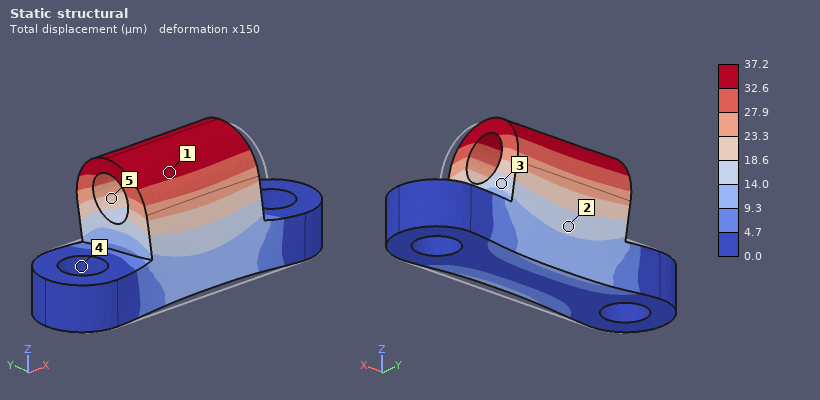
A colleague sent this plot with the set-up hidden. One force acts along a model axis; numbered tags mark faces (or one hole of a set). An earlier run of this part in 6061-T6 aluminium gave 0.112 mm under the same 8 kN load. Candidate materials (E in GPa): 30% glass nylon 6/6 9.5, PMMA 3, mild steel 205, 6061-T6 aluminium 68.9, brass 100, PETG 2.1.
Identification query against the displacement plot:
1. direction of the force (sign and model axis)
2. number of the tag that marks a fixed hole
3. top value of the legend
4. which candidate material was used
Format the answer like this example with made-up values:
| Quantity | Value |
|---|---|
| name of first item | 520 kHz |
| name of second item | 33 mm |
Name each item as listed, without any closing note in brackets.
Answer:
| Quantity | Value |
|---|---|
| direction of the force | +Y |
| number of the tag that marks a fixed hole | 4 |
| top value of the legend | 37.2 µm |
| which candidate material was used | mild steel |
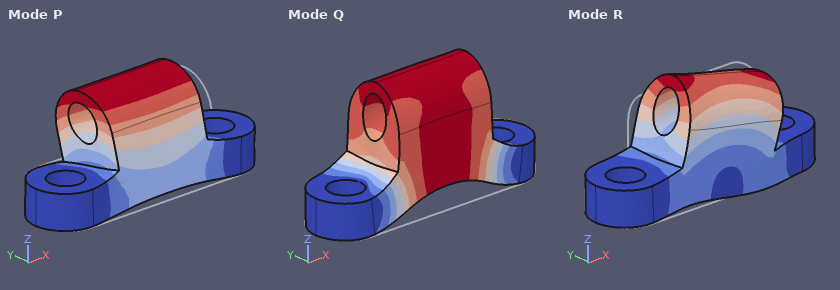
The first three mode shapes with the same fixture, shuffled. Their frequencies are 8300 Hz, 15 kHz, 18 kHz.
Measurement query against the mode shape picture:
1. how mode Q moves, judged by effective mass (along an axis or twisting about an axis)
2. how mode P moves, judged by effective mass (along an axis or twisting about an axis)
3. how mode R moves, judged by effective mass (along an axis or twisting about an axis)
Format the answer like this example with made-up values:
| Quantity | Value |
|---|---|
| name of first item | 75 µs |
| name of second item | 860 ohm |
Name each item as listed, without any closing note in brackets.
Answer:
| Quantity | Value |
|---|---|
| how mode Q moves, judged by effective mass | along Z |
| how mode P moves, judged by effective mass | along Y |
| how mode R moves, judged by effective mass | along X |
